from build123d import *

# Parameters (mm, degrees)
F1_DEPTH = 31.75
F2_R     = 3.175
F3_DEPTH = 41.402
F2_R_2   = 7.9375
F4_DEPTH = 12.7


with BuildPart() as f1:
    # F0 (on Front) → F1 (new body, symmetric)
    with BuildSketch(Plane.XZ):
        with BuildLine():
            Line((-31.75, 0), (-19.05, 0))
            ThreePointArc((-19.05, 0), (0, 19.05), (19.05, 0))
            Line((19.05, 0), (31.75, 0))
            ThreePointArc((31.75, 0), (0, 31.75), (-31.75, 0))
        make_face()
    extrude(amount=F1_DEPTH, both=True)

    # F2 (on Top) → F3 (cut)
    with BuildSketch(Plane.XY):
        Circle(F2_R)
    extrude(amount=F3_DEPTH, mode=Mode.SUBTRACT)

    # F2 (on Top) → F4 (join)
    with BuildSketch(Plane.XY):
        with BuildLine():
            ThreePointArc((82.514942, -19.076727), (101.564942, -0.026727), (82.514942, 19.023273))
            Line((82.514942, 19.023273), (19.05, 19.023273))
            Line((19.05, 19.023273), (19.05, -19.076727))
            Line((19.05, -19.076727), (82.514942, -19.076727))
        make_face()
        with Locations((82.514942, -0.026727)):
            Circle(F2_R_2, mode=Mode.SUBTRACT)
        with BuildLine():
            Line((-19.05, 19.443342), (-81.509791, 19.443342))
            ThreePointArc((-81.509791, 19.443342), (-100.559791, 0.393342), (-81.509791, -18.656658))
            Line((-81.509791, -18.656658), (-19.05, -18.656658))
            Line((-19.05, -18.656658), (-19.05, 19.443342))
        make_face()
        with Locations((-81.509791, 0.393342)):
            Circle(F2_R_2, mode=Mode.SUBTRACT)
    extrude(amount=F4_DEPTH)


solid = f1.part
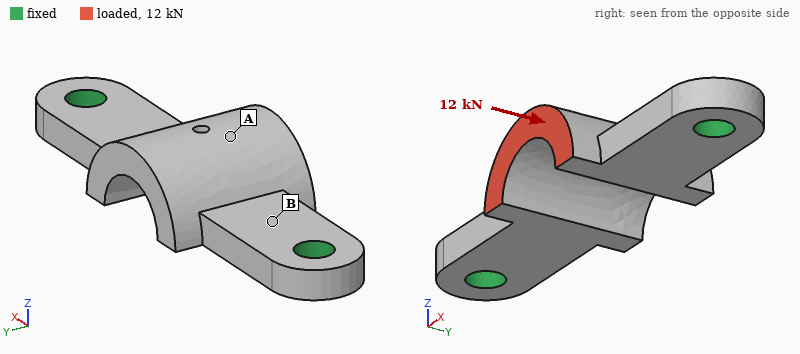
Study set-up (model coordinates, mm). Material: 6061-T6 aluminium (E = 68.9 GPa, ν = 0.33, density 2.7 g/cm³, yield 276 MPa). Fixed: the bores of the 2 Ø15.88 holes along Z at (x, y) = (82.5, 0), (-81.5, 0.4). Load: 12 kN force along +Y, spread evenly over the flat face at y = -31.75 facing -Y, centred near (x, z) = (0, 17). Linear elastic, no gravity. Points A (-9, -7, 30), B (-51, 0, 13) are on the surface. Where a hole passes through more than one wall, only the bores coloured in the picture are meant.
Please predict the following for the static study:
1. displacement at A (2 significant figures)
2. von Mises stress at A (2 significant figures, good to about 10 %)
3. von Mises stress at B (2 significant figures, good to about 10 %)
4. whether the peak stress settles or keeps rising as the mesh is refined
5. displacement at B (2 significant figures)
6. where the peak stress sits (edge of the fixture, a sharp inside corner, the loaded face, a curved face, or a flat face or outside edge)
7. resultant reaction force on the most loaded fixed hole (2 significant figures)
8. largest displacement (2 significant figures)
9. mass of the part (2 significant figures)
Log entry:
0.27 mm
21 MPa
93 MPa
keeps rising
0.063 mm
edge of the fixture
6.1 kN
0.35 mm
330 g
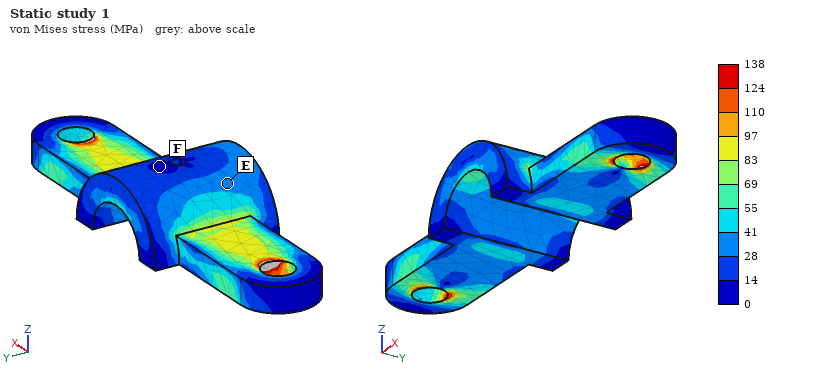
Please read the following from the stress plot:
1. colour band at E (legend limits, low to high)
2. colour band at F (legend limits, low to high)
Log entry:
28 to 41 MPa
0 to 14 MPa
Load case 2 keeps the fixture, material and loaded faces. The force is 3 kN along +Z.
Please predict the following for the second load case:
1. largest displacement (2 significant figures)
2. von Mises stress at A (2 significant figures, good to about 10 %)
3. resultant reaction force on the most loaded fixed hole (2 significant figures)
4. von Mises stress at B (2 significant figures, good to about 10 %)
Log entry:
0.23 mm
13 MPa
2.9 kN
45 MPa
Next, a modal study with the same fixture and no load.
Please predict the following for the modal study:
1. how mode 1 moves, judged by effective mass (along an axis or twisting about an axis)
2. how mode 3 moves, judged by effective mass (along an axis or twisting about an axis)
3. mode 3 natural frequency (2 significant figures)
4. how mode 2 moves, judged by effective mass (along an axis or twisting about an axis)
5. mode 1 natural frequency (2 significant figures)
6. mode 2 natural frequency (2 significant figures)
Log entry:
along Y
along Y
4700 Hz
along Z
2300 Hz
2500 Hz
